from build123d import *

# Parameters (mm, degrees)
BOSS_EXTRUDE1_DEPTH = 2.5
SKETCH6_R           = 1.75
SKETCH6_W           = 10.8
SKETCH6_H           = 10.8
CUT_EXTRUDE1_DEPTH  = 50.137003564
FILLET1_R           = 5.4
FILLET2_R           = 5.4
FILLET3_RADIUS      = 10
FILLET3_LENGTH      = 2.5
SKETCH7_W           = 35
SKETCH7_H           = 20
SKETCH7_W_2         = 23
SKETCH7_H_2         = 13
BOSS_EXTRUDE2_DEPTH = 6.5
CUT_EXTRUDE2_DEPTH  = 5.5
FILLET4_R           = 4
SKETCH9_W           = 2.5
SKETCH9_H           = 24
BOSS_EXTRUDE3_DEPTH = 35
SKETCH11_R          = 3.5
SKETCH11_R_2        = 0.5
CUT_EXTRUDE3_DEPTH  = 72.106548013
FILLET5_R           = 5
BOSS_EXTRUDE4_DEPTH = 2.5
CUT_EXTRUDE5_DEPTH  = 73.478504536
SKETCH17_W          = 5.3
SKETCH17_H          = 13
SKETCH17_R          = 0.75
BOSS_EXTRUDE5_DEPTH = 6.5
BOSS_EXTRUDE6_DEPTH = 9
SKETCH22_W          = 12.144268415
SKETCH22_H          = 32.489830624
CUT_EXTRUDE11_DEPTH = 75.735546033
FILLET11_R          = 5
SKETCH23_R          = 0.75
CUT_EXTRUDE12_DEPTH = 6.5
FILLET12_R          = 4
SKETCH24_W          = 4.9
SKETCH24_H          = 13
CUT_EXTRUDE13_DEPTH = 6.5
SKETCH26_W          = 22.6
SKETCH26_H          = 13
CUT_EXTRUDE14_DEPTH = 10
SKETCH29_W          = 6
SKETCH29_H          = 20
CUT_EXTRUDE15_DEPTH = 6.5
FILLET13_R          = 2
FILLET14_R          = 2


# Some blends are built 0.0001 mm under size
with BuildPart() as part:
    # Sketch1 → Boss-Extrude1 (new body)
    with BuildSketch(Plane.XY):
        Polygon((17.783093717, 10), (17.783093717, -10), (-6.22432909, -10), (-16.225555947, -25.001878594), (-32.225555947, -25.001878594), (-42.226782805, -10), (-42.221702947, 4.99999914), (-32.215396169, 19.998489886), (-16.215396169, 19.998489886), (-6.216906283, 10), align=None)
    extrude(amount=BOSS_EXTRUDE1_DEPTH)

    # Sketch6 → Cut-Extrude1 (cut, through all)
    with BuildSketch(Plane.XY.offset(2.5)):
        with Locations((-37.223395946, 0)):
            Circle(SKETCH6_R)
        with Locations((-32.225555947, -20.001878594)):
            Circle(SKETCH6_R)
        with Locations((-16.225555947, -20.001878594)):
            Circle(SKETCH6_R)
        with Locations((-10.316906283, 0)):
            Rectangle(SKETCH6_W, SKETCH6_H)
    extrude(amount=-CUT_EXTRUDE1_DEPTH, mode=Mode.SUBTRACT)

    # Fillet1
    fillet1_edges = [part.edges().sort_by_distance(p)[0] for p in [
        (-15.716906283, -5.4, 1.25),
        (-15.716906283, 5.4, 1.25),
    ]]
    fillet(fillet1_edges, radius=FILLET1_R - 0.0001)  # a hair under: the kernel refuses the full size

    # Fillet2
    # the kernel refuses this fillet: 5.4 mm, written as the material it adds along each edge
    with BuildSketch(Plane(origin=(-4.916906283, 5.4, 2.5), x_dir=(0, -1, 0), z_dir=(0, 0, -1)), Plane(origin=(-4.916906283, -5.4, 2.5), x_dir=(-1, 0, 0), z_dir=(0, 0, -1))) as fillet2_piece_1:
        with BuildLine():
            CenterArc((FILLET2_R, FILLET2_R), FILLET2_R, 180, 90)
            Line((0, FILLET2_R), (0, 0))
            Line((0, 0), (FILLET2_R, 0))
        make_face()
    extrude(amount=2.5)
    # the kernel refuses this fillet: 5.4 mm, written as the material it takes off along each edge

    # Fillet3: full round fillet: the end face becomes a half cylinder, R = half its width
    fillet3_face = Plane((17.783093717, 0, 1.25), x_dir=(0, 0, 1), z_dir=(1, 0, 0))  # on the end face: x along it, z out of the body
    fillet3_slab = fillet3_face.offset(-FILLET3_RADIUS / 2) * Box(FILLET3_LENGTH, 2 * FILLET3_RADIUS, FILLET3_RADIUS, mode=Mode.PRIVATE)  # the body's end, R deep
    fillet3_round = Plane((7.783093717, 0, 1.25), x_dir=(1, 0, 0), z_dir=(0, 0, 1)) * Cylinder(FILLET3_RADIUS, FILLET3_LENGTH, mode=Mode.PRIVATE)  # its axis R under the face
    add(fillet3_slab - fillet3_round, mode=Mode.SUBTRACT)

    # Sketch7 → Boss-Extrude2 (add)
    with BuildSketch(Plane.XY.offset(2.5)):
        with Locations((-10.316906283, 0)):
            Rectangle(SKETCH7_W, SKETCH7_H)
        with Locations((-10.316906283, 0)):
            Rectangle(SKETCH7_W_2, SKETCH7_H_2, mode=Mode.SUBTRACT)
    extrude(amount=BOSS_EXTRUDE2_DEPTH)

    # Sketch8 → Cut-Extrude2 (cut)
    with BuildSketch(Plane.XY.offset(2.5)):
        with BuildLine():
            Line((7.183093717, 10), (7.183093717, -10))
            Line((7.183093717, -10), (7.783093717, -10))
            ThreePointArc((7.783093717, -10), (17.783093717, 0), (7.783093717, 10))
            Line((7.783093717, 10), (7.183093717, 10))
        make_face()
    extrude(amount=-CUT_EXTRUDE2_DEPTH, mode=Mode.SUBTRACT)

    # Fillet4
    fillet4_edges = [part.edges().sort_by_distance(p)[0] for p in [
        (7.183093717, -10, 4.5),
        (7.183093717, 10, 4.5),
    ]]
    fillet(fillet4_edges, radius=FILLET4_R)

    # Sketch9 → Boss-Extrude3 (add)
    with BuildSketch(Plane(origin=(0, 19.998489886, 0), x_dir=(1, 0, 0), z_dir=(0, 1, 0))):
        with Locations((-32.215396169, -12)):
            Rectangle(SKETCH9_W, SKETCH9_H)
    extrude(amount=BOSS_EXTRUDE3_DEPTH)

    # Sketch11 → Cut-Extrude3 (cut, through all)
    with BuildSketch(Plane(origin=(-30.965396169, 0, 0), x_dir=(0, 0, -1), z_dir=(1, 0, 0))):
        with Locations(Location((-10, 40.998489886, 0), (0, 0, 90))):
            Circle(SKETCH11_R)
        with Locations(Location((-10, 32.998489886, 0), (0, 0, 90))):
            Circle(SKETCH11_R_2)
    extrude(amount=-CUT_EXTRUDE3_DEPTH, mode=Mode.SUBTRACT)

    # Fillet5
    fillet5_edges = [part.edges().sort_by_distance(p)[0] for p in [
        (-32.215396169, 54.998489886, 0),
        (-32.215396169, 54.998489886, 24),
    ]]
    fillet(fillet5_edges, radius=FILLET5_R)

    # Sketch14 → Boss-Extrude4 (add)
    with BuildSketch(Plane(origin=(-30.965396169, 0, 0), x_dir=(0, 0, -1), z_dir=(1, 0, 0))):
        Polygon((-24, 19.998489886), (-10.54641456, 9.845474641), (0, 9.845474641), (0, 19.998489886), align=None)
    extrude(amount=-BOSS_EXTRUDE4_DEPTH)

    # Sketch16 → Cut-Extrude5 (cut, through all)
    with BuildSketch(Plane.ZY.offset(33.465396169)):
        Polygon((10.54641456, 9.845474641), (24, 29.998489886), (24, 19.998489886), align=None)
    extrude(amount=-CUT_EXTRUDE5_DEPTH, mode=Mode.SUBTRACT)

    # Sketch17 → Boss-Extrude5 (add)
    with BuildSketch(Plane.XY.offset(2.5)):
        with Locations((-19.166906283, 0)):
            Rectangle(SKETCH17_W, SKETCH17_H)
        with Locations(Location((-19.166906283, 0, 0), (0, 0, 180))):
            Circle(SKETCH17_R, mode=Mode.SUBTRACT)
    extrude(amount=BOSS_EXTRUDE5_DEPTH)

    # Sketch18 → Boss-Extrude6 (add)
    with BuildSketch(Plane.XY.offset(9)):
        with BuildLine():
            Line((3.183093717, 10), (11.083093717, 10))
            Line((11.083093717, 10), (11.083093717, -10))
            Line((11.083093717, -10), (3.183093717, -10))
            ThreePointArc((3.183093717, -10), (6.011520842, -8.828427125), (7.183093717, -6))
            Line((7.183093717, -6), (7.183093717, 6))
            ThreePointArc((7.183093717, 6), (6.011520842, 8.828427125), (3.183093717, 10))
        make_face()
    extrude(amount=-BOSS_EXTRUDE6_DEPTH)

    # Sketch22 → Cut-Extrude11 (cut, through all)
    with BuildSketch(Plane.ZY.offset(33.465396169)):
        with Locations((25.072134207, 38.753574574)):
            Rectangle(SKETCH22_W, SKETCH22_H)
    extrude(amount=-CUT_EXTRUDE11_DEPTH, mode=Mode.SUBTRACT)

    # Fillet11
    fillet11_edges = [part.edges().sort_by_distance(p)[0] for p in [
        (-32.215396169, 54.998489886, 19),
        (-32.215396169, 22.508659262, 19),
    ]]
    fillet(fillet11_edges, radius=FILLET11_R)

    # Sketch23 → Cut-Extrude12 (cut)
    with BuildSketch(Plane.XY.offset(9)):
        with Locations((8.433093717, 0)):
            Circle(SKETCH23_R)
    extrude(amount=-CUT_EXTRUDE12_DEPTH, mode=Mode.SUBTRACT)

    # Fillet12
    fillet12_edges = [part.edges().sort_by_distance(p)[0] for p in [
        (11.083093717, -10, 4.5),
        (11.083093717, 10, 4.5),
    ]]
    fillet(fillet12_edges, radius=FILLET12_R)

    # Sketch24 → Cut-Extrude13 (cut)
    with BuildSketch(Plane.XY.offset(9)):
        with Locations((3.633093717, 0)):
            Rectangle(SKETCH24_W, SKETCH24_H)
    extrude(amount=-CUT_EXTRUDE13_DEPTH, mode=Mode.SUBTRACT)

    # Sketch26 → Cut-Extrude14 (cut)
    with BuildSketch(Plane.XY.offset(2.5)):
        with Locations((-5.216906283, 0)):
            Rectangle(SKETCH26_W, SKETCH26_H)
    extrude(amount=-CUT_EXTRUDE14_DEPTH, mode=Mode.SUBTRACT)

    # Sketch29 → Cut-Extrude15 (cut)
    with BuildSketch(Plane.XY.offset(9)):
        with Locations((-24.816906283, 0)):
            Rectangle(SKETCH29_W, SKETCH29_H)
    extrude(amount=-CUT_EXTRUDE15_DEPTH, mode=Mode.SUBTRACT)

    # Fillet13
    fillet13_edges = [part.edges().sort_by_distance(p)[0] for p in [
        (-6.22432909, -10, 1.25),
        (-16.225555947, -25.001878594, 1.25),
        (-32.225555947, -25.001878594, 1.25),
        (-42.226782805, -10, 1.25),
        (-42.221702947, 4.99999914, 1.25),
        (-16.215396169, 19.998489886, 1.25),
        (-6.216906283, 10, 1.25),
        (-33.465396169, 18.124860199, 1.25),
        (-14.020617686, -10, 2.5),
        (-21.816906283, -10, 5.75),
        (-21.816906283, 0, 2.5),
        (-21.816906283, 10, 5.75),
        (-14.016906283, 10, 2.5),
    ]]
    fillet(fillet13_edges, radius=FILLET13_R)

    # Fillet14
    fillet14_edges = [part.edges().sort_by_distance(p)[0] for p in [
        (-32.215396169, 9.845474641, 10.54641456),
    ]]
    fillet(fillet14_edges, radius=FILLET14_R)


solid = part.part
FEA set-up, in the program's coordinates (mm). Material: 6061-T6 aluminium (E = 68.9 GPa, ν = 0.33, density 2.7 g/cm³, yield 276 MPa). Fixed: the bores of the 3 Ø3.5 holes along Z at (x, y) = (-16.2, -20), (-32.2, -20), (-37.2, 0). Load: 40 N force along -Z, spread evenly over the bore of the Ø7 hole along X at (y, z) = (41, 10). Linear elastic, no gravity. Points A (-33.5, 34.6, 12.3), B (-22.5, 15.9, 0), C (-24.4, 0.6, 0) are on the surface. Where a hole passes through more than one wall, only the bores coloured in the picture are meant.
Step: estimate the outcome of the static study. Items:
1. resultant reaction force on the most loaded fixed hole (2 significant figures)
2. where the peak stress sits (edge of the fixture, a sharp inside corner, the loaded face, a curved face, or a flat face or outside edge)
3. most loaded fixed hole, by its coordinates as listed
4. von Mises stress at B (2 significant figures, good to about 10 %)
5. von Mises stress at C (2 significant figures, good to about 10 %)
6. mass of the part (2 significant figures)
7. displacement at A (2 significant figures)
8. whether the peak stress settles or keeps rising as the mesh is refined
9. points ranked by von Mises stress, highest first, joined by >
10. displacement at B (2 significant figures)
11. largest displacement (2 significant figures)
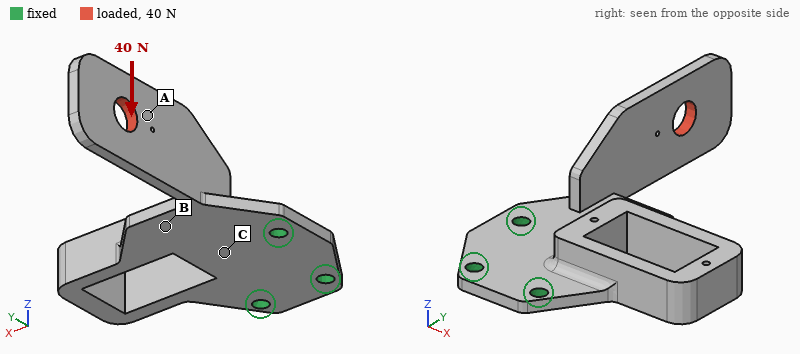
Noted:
83 N
edge of the fixture
(-37.2, 0)
26 MPa
15 MPa
20 g
0.22 mm
keeps rising
B > C > A
0.064 mm
0.37 mm
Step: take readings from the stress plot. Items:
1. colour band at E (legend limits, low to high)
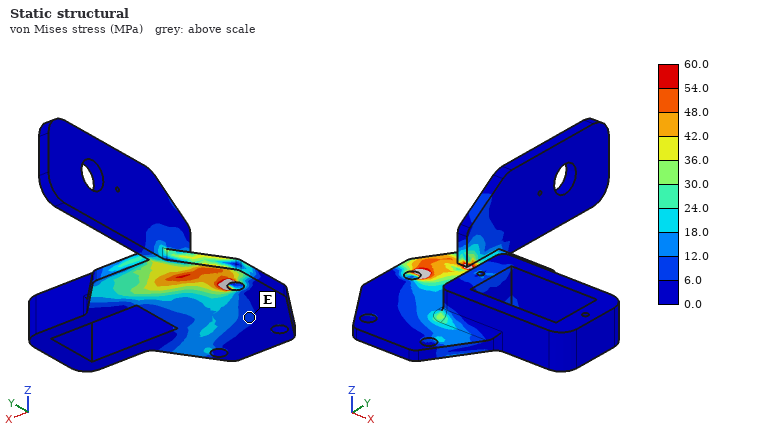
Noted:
6.0 to 12.0 MPa
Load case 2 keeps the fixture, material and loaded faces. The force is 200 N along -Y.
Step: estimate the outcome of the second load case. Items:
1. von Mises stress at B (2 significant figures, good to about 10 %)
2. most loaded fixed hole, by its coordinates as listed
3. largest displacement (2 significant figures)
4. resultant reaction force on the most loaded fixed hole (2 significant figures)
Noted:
36 MPa
(-37.2, 0)
0.46 mm
140 N
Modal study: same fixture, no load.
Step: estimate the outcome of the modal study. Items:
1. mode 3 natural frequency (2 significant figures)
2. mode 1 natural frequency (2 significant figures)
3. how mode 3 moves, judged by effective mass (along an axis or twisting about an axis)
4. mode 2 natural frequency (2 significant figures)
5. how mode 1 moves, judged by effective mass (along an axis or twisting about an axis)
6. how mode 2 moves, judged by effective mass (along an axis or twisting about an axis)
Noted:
1700 Hz
950 Hz
along Z
1100 Hz
along Z
along X
